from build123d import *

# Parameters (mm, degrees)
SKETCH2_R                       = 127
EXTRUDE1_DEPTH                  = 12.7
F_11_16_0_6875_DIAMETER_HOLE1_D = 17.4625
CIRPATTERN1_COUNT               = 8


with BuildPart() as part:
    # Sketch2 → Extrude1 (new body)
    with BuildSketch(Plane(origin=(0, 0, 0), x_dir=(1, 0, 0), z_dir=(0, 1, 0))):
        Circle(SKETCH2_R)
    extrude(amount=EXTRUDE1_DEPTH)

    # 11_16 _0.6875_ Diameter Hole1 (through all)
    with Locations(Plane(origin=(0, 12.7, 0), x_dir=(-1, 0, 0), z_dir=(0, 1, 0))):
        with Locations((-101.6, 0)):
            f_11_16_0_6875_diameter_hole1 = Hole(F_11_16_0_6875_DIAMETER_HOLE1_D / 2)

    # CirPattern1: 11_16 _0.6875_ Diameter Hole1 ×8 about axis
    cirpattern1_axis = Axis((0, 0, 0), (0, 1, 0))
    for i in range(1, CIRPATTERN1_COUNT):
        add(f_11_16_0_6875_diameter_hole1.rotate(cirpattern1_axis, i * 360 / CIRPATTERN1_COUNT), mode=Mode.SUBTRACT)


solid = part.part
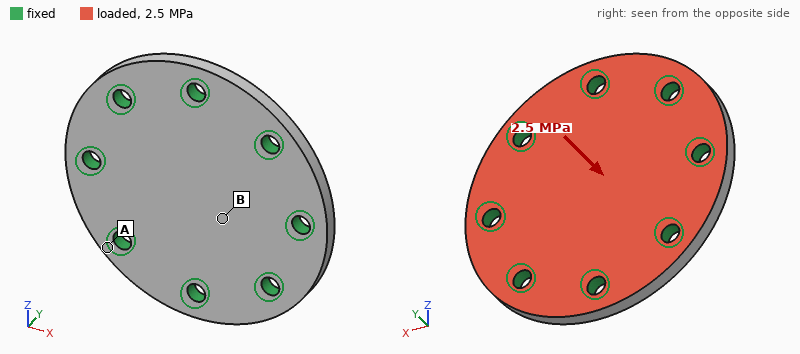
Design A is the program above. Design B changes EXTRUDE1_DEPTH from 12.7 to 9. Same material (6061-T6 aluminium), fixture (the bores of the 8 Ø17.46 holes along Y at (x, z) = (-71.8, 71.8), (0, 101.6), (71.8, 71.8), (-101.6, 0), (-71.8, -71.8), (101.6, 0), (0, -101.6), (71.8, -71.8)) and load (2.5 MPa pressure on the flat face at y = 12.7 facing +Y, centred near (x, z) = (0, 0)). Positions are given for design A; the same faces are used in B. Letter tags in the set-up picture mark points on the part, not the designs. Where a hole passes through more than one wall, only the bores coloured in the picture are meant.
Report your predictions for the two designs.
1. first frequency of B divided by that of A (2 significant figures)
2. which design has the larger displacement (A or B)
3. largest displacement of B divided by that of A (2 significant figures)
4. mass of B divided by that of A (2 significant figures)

0.74
B
2.6
0.71
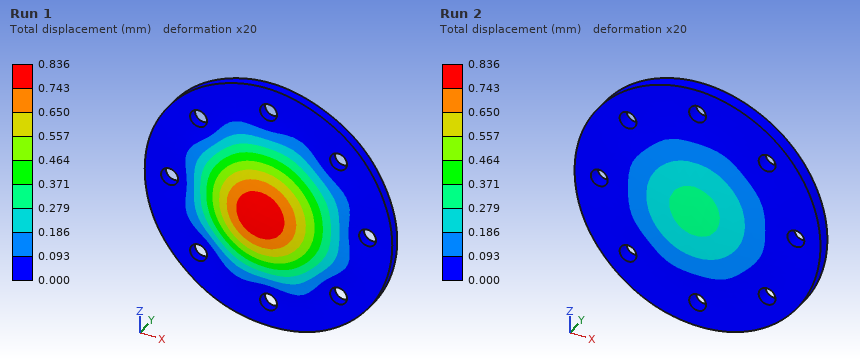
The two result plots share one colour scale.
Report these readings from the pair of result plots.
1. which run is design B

Run 1
